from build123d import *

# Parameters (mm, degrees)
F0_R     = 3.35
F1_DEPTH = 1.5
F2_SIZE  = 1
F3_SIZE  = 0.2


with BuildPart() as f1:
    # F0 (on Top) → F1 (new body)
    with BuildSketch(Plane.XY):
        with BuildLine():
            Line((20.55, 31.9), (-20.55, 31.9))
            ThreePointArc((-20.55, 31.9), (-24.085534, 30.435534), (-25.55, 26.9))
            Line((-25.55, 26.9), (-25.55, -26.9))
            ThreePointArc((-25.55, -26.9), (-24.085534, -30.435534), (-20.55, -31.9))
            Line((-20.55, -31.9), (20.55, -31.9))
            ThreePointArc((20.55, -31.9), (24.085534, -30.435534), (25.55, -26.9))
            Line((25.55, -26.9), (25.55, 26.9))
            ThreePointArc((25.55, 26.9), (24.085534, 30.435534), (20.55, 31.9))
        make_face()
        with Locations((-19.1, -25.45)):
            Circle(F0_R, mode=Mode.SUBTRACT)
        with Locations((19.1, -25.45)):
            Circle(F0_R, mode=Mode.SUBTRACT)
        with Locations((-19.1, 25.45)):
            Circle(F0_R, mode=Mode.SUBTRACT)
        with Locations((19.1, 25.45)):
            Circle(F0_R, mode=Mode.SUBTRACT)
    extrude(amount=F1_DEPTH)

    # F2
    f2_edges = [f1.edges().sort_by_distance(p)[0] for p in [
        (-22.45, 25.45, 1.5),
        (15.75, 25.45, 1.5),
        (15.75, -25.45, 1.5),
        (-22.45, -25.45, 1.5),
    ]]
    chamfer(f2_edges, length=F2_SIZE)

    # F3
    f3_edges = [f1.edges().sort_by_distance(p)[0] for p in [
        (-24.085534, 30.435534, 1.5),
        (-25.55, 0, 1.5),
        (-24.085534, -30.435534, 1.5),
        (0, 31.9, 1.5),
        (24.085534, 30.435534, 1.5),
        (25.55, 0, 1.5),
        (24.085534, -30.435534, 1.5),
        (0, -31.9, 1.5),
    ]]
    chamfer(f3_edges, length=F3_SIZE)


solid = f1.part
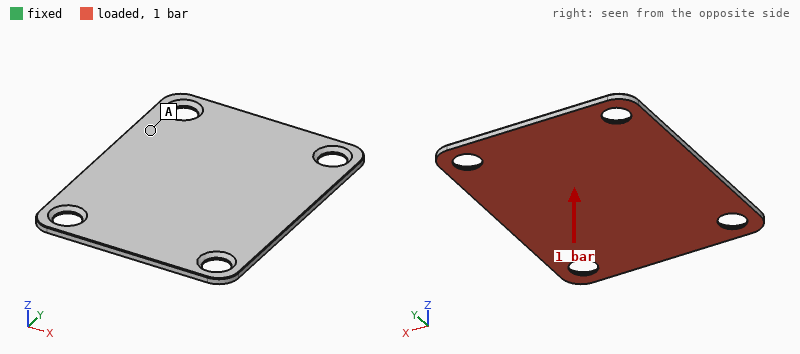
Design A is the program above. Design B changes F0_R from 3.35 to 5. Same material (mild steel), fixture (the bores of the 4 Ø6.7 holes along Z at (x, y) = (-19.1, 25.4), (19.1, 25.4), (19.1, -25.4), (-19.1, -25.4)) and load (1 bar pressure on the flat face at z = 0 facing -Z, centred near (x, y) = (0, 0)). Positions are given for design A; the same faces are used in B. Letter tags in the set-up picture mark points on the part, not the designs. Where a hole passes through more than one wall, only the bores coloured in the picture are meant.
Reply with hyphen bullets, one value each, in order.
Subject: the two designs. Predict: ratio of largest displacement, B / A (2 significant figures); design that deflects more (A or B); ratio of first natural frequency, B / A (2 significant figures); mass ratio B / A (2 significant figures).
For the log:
- 0.77
- A
- 1.2
- 0.94
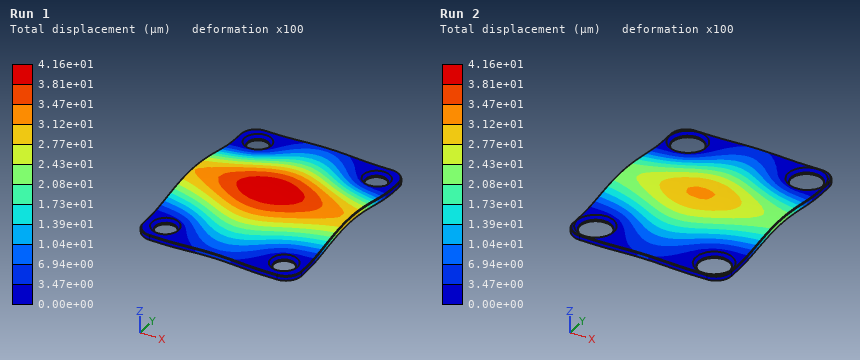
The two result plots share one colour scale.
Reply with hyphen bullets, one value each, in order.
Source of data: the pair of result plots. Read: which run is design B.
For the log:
- Run 2
